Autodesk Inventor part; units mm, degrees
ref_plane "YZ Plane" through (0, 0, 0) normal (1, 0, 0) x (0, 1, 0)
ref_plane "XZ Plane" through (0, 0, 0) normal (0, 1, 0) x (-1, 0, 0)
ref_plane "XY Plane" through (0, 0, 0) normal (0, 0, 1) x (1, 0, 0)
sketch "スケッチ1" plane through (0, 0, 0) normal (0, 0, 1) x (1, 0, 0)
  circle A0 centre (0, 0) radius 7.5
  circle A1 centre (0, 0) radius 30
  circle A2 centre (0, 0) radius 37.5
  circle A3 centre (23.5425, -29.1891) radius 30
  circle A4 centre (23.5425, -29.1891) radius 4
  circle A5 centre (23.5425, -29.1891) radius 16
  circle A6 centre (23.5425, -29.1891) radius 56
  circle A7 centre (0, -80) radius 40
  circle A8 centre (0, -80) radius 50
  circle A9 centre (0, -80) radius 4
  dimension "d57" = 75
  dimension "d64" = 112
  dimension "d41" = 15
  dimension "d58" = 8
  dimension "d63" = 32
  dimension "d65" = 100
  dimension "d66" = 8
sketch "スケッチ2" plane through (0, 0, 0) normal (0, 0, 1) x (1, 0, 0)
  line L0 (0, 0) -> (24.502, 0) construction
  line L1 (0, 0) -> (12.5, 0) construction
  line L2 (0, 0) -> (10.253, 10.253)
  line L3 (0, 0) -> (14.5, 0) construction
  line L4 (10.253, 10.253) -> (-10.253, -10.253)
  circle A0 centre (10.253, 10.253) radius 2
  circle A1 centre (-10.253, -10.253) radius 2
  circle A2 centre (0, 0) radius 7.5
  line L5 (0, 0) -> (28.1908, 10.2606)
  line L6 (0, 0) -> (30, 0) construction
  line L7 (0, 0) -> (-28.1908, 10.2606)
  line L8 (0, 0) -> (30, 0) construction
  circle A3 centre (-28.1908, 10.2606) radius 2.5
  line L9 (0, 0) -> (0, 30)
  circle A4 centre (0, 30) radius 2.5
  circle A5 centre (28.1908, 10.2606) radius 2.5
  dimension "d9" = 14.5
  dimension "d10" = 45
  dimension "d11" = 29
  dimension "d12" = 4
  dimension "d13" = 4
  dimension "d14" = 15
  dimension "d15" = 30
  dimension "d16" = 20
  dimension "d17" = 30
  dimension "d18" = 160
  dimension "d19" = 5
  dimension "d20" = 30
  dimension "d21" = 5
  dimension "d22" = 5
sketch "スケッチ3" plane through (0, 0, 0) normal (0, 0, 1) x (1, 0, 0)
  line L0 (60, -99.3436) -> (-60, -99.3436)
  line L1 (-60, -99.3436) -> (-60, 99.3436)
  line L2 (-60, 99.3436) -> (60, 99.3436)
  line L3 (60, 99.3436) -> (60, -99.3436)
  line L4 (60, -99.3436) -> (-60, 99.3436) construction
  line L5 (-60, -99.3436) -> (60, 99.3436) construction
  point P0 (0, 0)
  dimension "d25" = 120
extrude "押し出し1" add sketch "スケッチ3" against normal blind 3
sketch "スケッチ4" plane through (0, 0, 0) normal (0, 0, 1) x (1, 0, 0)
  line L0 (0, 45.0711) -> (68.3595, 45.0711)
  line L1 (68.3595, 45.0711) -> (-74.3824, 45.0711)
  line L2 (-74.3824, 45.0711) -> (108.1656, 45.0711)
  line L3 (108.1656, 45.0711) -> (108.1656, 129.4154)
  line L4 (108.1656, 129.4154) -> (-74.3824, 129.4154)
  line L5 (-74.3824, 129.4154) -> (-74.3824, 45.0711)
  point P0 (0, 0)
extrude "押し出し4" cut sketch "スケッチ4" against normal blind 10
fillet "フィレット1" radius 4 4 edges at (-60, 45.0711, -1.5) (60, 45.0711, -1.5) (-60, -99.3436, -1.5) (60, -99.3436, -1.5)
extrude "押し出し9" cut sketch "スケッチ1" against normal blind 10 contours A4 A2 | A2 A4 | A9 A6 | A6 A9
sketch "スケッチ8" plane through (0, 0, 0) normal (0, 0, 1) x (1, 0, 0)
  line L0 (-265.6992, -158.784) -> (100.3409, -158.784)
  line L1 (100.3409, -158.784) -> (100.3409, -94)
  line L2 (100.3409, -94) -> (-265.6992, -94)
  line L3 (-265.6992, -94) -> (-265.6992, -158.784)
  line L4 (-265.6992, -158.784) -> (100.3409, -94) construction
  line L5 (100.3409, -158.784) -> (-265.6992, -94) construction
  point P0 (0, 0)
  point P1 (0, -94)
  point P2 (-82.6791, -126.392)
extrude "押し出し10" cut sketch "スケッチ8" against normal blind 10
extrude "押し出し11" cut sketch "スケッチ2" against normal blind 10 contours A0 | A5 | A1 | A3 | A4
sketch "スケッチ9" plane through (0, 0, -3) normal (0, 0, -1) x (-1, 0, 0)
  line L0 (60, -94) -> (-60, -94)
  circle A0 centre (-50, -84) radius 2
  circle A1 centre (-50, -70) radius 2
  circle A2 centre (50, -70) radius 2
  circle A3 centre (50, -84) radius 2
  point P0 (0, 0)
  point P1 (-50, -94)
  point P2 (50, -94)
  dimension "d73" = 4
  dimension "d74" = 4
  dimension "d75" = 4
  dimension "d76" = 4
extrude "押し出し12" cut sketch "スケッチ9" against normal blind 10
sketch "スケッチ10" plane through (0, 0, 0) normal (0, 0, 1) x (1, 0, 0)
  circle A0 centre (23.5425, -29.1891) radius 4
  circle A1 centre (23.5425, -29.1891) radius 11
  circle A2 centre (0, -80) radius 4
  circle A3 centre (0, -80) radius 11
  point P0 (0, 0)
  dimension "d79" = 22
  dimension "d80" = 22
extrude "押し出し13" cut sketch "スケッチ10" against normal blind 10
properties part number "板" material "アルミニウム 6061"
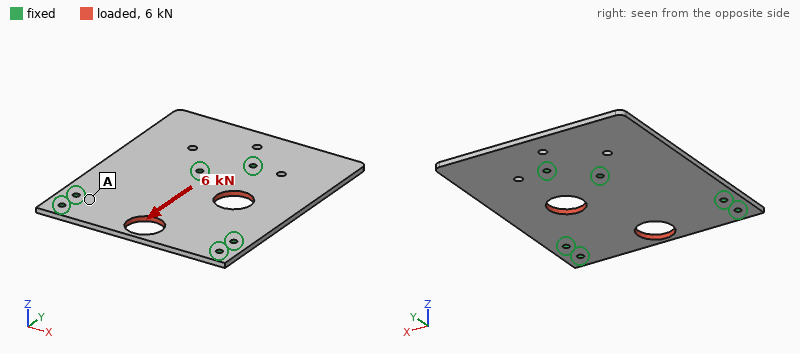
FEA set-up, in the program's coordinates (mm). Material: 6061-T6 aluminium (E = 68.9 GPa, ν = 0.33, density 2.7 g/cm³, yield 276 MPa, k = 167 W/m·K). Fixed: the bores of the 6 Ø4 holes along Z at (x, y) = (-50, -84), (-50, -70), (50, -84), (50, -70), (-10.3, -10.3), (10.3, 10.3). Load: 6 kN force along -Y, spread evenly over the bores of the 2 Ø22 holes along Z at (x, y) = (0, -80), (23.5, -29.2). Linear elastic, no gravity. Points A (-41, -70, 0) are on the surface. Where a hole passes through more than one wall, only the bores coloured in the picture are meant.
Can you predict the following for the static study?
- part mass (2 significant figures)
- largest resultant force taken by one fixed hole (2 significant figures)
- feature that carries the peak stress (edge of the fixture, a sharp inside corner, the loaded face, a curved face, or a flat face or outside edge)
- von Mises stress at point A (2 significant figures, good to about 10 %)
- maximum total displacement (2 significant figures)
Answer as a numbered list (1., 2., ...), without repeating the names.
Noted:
1. 130 g
2. 1.6 kN
3. a flat face or outside edge
4. 14 MPa
5. 44 µm
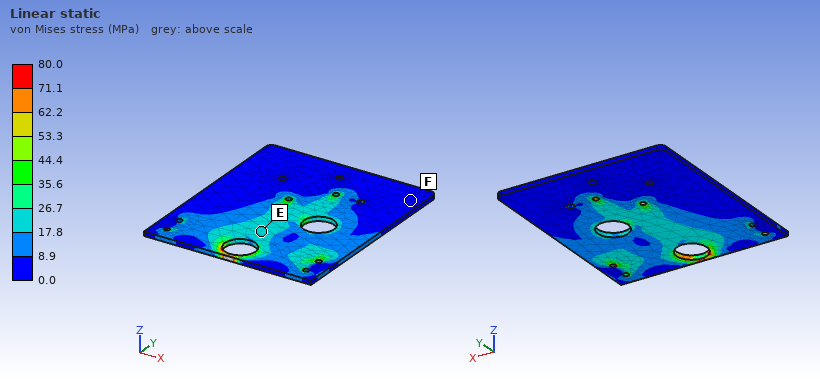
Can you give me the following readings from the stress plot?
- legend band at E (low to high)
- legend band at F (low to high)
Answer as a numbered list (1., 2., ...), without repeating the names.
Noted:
1. 17.8 to 26.7 MPa
2. 0.0 to 8.9 MPa
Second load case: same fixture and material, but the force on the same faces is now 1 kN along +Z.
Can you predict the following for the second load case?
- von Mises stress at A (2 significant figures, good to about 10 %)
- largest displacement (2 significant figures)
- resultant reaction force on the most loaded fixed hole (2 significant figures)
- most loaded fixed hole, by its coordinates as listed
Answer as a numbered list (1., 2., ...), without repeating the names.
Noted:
1. 63 MPa
2. 0.61 mm
3. 330 N
4. (50, -70)
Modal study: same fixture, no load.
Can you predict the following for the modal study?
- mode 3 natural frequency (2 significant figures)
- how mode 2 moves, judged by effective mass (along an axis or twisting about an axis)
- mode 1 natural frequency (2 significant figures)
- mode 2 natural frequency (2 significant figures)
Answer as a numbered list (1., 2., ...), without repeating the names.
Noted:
1. 1500 Hz
2. along Z
3. 730 Hz
4. 970 Hz
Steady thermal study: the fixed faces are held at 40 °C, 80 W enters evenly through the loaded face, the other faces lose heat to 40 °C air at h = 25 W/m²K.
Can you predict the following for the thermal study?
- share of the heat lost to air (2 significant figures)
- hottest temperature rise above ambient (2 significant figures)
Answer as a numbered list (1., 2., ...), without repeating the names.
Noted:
1. 14 %
2. 56 K
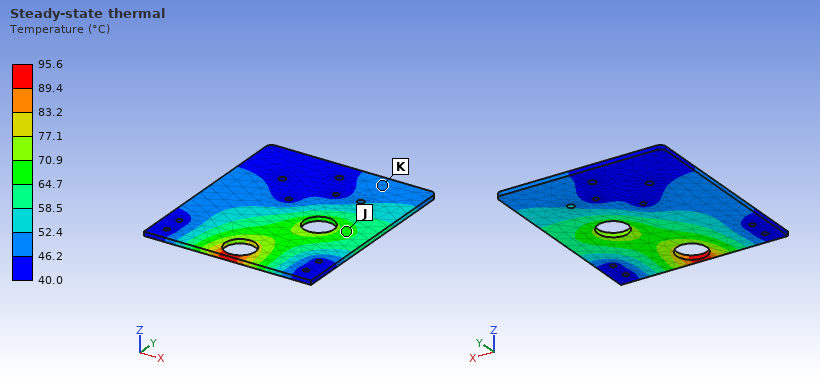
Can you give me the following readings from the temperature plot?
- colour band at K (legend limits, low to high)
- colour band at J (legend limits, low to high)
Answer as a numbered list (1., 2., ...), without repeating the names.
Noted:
1. 46.2 to 52.4 °C
2. 64.7 to 70.9 °C
